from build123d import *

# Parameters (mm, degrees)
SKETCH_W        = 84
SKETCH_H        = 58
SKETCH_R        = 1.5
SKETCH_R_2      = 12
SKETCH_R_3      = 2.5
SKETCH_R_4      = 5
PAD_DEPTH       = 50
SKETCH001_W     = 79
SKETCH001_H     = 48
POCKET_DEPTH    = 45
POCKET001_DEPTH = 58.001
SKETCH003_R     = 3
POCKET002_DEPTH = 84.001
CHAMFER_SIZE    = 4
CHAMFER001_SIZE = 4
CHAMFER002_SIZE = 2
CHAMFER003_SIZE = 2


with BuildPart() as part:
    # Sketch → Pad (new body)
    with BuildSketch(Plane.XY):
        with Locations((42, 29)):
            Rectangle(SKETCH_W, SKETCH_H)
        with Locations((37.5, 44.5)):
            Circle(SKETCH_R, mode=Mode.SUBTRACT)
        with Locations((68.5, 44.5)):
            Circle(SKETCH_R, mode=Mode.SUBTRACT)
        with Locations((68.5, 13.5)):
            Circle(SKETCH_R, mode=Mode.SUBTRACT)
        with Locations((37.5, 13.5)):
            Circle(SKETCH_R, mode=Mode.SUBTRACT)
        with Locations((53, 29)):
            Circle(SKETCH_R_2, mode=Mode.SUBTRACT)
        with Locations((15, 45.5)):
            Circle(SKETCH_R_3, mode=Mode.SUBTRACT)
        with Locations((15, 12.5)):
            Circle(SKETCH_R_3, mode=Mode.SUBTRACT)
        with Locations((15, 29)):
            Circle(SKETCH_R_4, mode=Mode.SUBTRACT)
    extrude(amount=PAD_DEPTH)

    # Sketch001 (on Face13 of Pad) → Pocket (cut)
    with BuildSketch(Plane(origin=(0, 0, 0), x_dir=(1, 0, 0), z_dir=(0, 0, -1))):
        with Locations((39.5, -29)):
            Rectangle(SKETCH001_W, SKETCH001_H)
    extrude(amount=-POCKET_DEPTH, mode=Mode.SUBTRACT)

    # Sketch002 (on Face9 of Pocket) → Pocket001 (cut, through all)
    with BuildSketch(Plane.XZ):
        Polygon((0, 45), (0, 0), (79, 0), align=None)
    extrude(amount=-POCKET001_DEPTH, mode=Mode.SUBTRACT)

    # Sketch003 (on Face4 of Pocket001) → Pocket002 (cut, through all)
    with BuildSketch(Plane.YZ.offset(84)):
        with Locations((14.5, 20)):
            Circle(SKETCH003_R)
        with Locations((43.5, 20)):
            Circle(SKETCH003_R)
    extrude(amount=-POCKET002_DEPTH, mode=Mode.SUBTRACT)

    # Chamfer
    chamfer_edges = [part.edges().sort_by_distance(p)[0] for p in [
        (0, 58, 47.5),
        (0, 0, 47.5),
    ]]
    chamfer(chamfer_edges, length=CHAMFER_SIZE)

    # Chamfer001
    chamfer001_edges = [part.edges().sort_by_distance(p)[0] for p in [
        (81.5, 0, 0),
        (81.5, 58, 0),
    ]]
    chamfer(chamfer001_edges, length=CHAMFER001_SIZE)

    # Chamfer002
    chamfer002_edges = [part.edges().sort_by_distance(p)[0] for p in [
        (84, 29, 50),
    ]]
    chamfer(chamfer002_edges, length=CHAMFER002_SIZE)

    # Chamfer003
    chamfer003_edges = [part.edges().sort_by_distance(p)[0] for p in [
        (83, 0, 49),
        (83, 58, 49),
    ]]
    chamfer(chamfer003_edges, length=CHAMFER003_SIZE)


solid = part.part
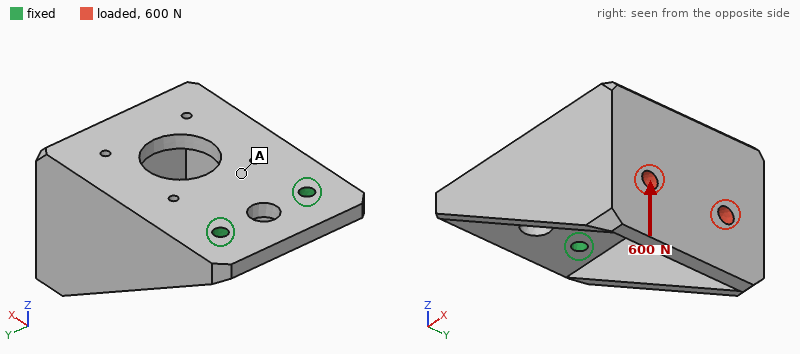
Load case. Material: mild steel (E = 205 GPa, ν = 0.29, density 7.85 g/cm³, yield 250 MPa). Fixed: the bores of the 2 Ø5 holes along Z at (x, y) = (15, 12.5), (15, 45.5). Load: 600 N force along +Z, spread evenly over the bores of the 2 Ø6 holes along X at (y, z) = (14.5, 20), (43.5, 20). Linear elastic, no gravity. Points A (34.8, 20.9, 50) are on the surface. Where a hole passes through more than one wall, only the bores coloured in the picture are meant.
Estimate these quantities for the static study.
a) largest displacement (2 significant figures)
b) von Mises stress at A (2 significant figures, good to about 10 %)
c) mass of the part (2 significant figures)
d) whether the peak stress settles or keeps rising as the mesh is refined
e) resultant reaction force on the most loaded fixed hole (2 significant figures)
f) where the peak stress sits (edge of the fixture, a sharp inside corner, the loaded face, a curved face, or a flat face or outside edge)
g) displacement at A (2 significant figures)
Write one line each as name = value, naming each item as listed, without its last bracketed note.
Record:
largest displacement = 0.17 mm
von Mises stress at A = 23 MPa
mass of the part = 400 g
whether the peak stress settles or keeps rising as the mesh is refined = keeps rising
resultant reaction force on the most loaded fixed hole = 320 N
where the peak stress sits = edge of the fixture
displacement at A = 0.029 mm
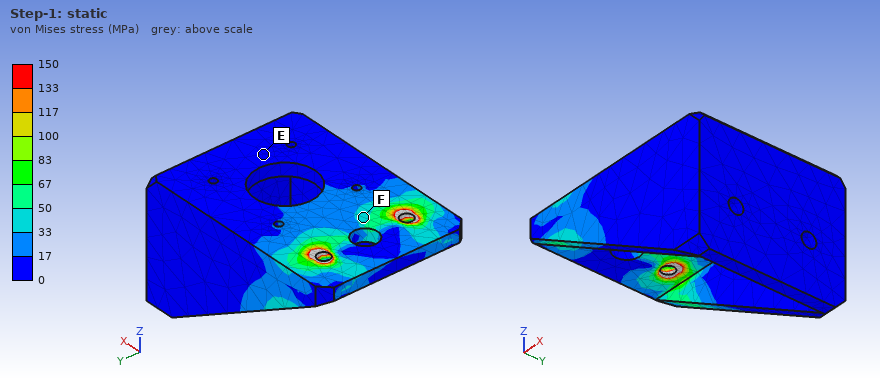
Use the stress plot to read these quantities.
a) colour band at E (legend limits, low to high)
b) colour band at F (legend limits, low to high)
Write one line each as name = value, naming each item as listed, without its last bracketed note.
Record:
colour band at E = 0 to 17 MPa
colour band at F = 33 to 50 MPa
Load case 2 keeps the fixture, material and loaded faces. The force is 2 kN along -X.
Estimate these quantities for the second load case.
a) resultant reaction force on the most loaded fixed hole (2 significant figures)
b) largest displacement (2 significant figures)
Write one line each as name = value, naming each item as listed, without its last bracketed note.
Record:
resultant reaction force on the most loaded fixed hole = 1.0 kN
largest displacement = 0.25 mm
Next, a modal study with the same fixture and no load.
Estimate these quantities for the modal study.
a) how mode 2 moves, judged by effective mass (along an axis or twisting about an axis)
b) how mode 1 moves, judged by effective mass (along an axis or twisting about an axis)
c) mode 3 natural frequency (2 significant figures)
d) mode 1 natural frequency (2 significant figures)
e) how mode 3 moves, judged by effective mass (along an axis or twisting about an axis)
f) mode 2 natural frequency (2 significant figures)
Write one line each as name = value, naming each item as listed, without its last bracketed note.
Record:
how mode 2 moves, judged by effective mass = along Y
how mode 1 moves, judged by effective mass = along Z
mode 3 natural frequency = 3400 Hz
mode 1 natural frequency = 700 Hz
how mode 3 moves, judged by effective mass = along Y
mode 2 natural frequency = 1100 Hz
